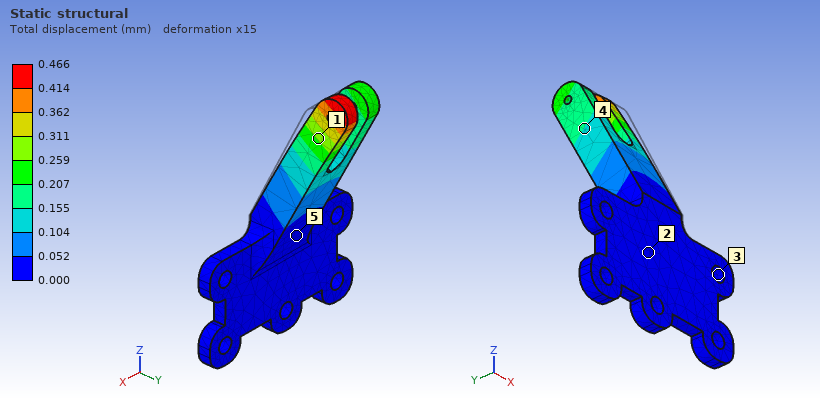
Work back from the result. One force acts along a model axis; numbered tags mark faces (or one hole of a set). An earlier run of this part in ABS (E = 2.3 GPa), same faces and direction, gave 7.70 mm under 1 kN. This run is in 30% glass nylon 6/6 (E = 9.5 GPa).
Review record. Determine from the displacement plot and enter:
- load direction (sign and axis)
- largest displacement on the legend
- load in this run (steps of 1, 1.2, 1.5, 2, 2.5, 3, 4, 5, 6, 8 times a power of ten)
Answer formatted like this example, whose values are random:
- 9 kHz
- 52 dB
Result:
- -X
- 0.466 mm
- 250 N
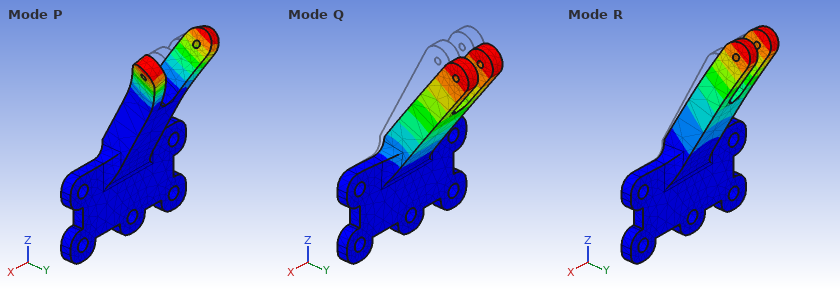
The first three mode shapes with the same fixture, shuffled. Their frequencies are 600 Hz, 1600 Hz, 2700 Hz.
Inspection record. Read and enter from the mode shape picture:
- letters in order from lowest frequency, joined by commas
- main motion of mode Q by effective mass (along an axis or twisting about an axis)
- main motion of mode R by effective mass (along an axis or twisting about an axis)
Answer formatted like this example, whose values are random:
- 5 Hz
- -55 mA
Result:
- Q, R, P
- along Y
- along X
